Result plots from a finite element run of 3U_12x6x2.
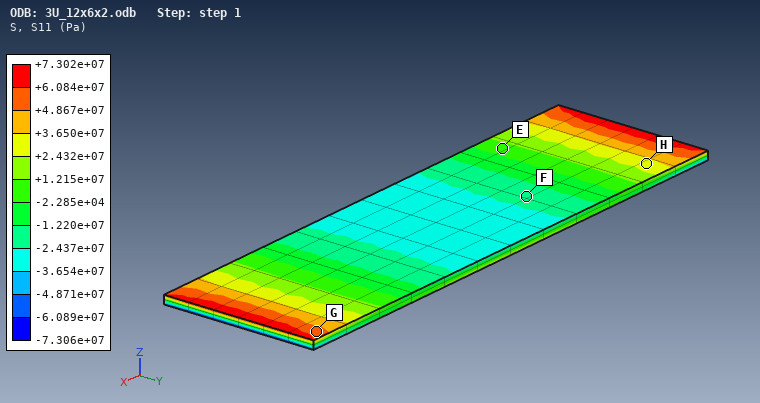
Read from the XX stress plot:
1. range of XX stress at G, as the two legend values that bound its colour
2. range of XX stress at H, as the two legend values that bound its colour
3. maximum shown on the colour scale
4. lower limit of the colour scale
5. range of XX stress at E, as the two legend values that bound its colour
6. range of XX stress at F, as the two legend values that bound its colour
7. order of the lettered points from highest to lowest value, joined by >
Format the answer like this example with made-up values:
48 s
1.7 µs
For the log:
+4.867e+07 to +6.084e+07 Pa
+2.432e+07 to +3.650e+07 Pa
+7.302e+07 Pa
-7.306e+07 Pa
-2.285e+04 to +1.215e+07 Pa
-2.437e+07 to -1.220e+07 Pa
G > H > E > F
